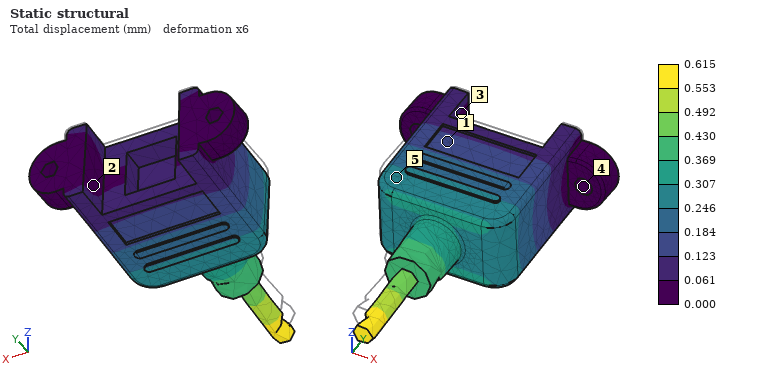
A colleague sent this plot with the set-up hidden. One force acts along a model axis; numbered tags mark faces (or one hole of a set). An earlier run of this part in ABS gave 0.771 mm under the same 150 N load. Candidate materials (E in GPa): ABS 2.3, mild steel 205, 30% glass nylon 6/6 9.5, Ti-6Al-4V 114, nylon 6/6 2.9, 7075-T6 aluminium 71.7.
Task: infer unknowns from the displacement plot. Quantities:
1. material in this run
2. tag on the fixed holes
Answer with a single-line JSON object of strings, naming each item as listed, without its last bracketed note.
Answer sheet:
{"material in this run": "nylon 6/6", "tag on the fixed holes": "4"}
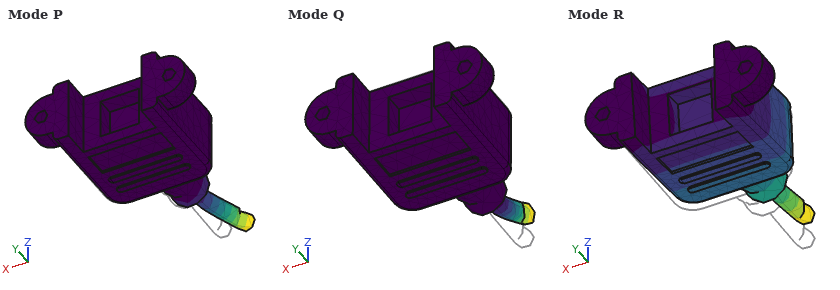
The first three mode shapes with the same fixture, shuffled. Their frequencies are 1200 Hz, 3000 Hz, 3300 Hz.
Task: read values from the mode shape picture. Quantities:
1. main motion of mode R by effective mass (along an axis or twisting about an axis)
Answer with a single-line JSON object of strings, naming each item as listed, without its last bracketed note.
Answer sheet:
{"main motion of mode R by effective mass": "along Z"}
